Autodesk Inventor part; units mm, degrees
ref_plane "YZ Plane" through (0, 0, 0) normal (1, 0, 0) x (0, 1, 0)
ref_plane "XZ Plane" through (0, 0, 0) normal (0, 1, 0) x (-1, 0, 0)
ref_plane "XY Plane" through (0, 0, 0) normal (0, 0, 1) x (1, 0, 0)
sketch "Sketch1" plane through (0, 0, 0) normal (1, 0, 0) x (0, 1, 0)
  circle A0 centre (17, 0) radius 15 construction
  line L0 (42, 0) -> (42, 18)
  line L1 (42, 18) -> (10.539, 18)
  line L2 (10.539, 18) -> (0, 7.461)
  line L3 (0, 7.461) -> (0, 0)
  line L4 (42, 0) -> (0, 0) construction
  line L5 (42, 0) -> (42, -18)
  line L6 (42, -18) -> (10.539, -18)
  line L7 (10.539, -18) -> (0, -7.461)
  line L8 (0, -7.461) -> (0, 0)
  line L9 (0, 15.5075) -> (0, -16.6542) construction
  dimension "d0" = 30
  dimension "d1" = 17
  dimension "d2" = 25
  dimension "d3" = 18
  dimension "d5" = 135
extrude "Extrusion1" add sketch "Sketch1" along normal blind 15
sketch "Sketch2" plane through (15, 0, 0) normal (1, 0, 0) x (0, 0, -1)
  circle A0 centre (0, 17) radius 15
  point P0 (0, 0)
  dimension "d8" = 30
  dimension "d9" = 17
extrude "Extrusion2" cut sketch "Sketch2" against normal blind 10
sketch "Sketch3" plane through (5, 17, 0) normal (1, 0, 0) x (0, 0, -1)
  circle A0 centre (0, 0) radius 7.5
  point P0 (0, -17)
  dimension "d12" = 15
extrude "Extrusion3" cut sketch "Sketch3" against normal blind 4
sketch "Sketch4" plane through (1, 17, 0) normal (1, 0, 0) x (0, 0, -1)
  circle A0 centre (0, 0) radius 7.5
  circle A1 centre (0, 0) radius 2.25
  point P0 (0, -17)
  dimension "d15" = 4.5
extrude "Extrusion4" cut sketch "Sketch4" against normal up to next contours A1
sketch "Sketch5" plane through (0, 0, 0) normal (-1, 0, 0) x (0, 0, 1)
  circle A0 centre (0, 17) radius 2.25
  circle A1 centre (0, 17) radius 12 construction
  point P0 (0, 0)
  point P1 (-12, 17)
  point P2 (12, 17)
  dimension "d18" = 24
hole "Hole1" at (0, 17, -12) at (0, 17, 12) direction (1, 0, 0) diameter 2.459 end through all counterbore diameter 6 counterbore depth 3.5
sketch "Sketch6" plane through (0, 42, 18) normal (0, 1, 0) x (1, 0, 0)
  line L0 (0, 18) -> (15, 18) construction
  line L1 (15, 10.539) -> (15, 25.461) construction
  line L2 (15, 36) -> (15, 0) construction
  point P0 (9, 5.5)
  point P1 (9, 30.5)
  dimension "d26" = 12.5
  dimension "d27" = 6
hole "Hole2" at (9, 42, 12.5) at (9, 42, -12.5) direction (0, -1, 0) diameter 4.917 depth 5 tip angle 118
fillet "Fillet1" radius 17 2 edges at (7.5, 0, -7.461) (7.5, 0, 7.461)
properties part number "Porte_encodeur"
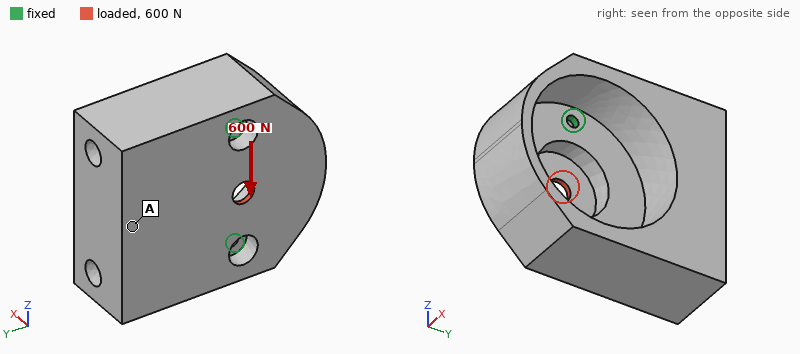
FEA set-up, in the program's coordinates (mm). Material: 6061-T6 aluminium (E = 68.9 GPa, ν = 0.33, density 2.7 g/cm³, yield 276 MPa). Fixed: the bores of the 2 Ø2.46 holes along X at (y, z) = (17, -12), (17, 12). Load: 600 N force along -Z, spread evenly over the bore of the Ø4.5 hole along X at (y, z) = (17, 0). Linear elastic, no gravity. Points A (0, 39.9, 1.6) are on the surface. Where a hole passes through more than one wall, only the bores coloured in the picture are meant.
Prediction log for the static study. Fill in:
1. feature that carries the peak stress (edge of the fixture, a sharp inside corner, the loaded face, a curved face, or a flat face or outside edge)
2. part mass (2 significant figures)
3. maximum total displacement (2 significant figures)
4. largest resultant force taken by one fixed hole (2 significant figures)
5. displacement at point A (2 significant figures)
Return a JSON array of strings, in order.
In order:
["the loaded face", "34 g", "6.3 µm", "310 N", "2.0 µm"]
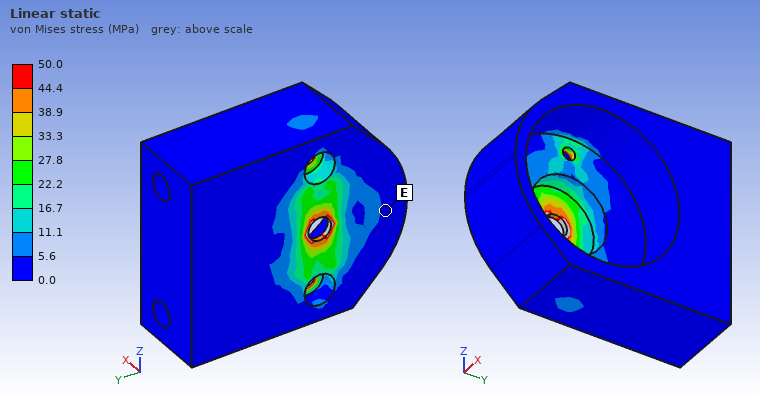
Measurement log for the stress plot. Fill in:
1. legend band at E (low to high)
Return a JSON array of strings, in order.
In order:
["0.0 to 5.6 MPa"]
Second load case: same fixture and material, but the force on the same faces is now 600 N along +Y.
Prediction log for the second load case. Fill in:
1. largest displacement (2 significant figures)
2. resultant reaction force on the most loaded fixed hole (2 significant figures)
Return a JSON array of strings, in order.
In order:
["89 µm", "300 N"]
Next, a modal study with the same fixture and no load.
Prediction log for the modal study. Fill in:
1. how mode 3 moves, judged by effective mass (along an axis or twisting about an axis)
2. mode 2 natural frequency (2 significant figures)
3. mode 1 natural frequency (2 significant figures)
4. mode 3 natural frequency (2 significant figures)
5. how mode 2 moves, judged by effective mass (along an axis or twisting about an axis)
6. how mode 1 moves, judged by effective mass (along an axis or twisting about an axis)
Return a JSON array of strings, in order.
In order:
["along Z", "7900 Hz", "1500 Hz", "11 kHz", "along Z", "along X"]
